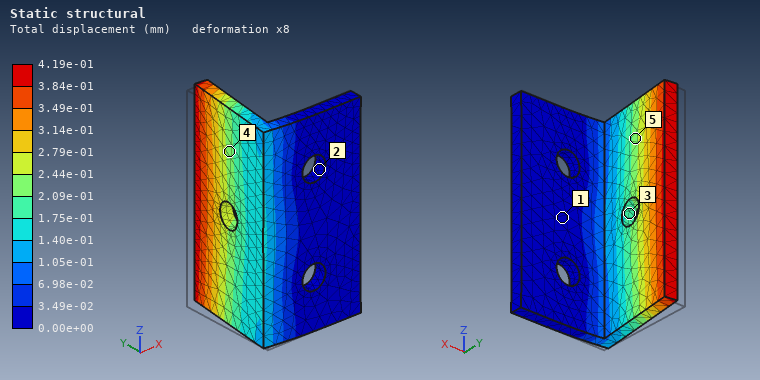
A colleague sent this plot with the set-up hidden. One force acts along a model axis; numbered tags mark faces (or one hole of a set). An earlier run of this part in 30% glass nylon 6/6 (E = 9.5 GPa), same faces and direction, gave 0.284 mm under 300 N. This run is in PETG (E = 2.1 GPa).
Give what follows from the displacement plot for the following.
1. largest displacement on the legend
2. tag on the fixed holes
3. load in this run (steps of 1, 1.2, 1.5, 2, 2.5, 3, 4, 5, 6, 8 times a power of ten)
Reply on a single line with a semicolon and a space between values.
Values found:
4.19e-01 mm; 2; 100 N
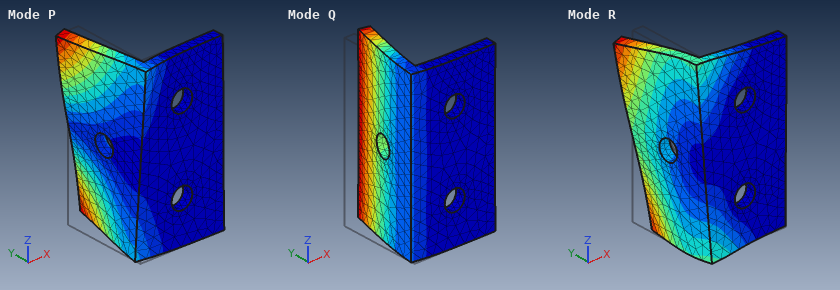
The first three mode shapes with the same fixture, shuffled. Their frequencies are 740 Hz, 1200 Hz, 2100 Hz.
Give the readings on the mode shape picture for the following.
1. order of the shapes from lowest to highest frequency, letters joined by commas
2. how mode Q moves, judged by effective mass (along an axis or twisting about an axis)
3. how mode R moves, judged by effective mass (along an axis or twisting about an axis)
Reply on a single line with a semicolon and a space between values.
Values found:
Q, P, R; along X; along Z
